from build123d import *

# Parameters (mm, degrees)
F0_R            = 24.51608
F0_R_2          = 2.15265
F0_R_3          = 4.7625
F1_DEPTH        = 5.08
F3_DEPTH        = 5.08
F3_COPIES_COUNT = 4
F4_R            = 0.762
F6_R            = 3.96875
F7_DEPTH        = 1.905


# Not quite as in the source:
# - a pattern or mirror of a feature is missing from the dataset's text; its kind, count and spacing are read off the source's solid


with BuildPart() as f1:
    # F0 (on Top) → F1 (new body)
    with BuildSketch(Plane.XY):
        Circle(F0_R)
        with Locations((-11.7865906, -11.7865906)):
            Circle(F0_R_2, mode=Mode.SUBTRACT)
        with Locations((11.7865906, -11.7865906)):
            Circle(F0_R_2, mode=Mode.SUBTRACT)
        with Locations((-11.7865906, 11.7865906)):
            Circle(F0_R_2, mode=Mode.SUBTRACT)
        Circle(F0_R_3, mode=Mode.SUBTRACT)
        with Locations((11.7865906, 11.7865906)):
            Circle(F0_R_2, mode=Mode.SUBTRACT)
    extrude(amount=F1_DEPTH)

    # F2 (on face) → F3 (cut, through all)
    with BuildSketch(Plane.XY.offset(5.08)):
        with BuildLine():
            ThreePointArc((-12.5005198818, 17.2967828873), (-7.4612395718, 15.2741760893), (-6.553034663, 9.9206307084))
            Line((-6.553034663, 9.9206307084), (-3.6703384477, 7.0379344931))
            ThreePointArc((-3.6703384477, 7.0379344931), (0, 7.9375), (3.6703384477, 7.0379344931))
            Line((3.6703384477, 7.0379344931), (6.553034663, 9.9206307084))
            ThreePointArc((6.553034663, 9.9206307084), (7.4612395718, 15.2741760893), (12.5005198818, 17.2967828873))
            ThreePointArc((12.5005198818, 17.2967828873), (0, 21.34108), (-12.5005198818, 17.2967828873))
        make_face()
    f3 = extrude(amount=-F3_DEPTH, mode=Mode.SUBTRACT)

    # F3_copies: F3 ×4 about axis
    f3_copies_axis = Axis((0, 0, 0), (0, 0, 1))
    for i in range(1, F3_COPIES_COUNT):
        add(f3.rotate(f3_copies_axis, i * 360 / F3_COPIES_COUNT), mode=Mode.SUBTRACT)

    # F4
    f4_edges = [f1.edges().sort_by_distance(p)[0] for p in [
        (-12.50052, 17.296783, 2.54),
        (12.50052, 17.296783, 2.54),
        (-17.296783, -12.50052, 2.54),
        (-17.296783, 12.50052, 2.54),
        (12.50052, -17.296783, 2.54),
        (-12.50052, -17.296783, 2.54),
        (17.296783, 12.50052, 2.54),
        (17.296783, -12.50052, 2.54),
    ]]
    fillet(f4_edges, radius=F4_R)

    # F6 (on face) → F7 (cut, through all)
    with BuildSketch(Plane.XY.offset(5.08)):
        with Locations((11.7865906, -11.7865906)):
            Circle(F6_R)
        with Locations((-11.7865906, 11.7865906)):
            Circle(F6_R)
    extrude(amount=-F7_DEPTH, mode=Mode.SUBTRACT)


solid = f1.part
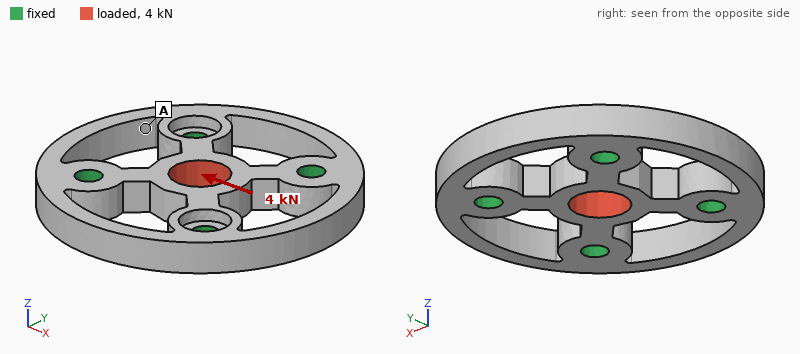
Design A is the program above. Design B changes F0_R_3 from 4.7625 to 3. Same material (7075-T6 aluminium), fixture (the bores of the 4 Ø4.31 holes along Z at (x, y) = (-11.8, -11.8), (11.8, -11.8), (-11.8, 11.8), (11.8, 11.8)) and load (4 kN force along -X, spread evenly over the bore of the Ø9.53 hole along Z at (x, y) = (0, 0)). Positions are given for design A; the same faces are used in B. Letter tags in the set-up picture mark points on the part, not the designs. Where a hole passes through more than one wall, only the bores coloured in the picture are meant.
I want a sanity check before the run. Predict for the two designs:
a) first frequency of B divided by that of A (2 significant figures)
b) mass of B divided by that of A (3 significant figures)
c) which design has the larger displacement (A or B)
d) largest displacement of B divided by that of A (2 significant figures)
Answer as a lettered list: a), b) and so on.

a) 1.0
b) 1.05
c) A
d) 0.76
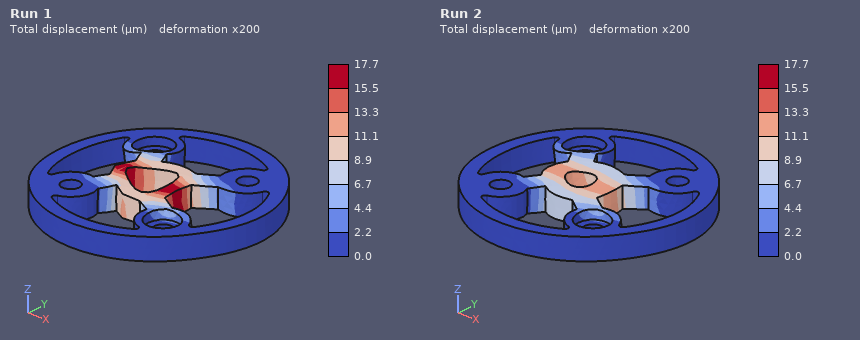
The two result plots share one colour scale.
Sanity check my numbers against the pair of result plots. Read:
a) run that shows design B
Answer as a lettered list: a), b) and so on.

a) Run 2
